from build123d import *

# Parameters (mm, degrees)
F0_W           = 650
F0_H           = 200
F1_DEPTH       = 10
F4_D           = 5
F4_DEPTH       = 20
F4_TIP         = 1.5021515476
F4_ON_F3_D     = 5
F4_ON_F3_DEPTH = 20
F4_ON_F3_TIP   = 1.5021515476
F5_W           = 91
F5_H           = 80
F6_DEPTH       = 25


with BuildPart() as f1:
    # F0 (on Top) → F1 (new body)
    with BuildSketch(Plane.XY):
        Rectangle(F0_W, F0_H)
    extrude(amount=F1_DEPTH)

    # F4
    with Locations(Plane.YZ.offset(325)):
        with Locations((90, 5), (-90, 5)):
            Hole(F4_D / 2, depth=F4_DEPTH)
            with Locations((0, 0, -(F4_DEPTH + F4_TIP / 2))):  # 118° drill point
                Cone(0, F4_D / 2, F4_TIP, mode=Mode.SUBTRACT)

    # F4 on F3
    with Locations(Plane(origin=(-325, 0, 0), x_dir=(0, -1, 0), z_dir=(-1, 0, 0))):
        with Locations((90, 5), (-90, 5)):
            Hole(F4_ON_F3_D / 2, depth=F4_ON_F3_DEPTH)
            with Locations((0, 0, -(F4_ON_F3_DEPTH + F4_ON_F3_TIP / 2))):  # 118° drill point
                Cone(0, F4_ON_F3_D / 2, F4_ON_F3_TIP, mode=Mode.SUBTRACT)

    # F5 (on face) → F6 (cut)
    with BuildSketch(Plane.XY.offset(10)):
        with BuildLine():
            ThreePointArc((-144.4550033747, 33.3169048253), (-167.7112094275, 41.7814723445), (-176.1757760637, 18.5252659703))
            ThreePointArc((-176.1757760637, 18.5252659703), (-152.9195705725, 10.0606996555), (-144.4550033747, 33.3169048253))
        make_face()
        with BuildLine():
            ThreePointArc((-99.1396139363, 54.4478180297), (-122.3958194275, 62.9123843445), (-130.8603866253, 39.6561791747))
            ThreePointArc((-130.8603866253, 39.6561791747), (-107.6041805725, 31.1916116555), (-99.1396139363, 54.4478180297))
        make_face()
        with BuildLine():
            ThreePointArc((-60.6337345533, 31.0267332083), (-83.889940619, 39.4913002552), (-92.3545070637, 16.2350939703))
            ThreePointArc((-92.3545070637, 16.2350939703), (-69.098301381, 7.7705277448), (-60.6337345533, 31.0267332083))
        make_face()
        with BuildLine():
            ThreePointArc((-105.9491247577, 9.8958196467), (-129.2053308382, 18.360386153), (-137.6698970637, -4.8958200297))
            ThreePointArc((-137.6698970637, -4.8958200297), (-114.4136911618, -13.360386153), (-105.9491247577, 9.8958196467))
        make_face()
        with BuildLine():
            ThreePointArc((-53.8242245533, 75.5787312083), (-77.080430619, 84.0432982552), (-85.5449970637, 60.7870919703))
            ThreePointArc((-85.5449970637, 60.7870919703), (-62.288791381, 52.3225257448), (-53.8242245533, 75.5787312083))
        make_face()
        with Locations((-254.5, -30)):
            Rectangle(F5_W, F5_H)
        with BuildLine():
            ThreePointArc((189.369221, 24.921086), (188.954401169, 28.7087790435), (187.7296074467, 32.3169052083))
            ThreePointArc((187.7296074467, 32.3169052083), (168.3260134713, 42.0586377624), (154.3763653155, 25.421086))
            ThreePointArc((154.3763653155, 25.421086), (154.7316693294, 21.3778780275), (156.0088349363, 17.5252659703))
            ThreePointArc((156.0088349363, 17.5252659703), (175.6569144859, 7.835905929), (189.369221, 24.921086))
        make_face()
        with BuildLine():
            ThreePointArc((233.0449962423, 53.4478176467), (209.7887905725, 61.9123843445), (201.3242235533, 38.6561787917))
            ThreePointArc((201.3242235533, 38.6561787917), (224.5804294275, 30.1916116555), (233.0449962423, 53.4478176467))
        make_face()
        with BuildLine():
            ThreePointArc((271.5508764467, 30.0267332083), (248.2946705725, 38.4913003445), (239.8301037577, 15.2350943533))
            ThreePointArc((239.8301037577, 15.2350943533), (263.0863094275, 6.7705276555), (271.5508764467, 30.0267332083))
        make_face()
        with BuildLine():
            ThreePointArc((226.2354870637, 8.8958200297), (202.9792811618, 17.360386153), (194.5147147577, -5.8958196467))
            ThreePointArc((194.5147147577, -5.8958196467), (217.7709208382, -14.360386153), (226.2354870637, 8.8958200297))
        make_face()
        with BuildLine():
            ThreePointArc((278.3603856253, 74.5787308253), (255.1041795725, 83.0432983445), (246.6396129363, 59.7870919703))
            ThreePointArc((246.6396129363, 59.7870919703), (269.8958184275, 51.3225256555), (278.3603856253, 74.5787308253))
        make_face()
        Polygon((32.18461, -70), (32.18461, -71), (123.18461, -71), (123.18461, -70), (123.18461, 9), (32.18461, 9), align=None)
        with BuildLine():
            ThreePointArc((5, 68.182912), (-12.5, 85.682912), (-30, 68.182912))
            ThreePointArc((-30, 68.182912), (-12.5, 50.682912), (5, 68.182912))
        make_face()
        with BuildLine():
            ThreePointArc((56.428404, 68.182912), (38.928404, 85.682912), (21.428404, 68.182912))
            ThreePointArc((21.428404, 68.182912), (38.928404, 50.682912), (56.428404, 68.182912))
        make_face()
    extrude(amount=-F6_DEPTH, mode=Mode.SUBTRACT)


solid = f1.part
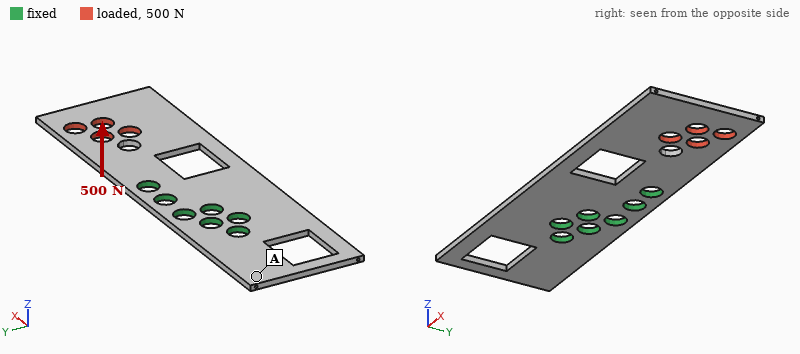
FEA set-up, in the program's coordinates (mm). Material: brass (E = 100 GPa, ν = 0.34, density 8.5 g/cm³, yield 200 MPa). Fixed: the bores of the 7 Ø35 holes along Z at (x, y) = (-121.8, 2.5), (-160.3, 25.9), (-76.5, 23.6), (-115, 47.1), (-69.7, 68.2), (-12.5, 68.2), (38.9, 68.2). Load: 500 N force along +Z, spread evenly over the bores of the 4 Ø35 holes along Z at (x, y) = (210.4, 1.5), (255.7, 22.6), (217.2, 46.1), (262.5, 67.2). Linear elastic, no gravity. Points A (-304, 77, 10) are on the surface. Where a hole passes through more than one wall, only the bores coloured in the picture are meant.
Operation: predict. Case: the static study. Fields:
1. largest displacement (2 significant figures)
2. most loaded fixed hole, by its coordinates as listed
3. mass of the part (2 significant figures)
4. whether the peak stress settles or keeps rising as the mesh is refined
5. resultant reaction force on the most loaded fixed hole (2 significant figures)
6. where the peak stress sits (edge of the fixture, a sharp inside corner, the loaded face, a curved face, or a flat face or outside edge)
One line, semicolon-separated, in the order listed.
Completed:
2.0 mm; (38.9, 68.2); 8.8 kg; keeps rising; 750 N; edge of the fixture
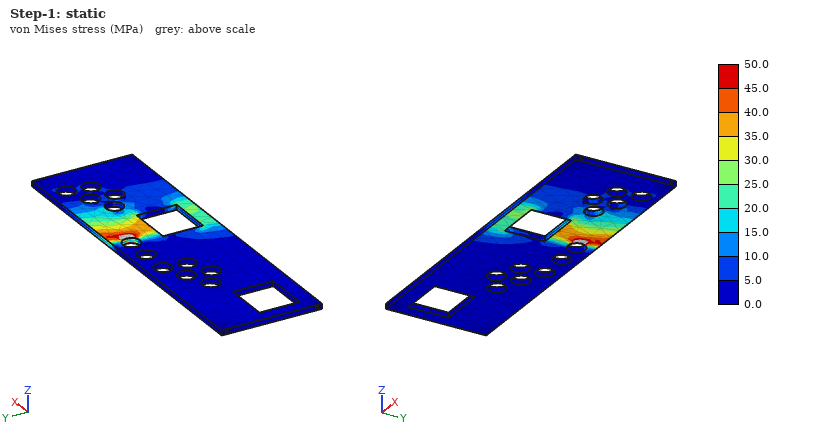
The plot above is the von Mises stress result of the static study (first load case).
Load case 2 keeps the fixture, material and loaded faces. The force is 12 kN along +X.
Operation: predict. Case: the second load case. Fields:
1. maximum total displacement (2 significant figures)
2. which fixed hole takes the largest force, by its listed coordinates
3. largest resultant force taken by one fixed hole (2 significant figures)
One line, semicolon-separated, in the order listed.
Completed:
34 µm; (38.9, 68.2); 8.6 kN
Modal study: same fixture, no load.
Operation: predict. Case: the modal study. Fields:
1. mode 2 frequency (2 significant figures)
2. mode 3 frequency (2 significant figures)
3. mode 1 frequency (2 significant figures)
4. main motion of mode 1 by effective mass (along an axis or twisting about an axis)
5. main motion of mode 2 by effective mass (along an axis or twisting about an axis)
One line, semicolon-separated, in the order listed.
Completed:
160 Hz; 200 Hz; 56 Hz; along Z; twisting about X
